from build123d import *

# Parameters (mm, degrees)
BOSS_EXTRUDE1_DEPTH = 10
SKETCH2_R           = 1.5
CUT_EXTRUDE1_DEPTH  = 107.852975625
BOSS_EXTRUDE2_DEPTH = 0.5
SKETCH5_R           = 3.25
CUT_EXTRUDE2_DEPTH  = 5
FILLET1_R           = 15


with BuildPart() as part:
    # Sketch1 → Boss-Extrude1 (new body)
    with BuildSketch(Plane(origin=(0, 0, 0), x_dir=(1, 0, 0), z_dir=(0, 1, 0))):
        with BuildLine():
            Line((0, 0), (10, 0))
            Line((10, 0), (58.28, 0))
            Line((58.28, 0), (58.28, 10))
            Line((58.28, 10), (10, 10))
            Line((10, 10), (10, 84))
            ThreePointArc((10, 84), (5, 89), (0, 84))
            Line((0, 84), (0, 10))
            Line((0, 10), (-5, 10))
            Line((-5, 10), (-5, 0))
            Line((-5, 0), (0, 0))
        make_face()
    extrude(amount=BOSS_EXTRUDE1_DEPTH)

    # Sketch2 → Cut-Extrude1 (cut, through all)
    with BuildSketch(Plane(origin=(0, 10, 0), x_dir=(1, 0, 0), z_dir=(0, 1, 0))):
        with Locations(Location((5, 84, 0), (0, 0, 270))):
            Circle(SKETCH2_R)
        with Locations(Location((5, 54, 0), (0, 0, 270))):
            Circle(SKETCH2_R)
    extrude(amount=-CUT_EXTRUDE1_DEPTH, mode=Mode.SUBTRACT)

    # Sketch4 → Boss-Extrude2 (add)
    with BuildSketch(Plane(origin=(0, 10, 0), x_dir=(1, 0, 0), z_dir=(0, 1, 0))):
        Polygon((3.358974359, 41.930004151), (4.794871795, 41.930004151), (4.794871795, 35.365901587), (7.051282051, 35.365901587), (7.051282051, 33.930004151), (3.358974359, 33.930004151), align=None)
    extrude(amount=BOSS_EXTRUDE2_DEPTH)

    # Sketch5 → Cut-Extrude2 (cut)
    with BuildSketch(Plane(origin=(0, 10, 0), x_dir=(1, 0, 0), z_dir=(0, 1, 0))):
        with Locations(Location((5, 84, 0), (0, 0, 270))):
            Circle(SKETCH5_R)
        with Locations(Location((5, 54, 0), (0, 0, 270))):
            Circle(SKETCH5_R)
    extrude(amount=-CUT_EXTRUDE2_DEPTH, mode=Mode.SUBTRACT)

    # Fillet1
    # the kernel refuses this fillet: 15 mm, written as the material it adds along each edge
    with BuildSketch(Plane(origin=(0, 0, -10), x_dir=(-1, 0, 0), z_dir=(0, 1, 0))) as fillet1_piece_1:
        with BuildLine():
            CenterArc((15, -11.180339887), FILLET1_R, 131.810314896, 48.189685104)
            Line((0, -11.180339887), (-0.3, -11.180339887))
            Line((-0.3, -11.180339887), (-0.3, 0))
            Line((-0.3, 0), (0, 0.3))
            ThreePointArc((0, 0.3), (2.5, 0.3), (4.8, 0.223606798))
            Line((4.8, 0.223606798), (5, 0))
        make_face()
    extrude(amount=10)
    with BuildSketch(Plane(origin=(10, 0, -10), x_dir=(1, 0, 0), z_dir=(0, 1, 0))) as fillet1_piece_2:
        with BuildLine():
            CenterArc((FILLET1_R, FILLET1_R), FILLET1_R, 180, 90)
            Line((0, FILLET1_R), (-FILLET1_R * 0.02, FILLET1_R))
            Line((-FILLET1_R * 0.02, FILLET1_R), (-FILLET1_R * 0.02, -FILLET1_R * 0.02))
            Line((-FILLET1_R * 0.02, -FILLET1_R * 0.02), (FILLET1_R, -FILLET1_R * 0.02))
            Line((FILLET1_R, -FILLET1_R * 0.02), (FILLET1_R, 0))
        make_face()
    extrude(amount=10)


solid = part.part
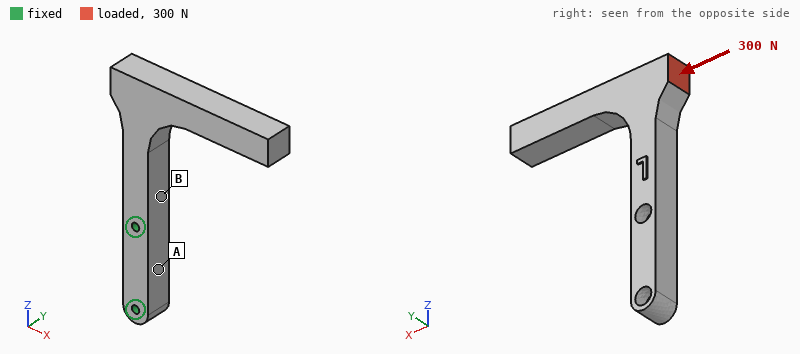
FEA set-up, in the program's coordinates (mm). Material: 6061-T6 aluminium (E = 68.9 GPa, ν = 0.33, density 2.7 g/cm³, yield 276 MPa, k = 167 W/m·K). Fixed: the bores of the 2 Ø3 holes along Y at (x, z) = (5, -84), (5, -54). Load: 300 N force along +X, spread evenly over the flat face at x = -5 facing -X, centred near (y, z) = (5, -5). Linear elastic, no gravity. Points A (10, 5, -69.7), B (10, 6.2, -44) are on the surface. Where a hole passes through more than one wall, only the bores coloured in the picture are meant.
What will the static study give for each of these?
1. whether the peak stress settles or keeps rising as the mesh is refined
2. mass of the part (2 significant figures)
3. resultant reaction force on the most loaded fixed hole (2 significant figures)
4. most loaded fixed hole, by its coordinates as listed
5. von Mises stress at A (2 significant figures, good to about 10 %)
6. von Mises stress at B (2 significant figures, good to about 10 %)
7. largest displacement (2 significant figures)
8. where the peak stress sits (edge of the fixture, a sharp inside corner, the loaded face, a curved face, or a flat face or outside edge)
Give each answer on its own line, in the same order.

keeps rising
39 g
620 N
(5, -54)
20 MPa
70 MPa
0.53 mm
edge of the fixture
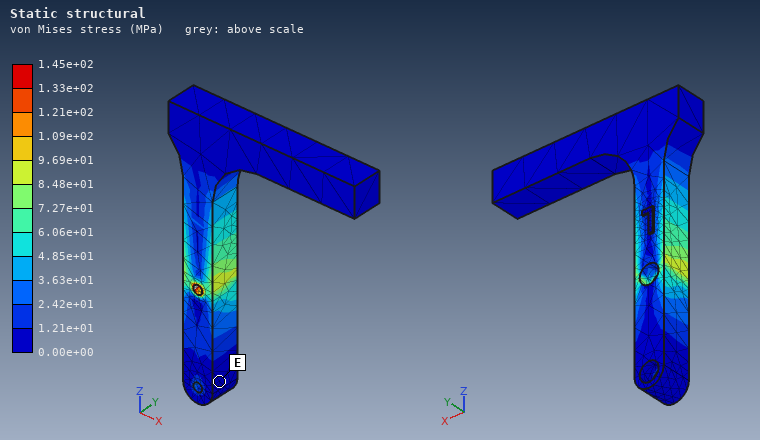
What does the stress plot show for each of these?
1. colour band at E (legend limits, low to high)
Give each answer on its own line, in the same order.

0.00e+00 to 1.21e+01 MPa
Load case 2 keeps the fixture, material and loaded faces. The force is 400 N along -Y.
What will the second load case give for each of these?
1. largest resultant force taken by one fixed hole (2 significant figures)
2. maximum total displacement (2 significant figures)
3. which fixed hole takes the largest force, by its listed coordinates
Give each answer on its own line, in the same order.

1.1 kN
0.52 mm
(5, -54)
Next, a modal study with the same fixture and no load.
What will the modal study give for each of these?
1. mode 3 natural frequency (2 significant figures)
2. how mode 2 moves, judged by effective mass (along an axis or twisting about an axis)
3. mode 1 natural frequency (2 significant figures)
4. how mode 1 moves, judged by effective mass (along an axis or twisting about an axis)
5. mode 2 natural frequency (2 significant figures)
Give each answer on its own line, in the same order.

2000 Hz
along X
860 Hz
along Y
910 Hz
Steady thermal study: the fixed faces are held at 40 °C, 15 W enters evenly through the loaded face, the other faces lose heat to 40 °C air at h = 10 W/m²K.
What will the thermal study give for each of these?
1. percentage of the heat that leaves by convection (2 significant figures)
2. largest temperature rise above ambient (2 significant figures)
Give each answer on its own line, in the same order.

8.6 %
44 K
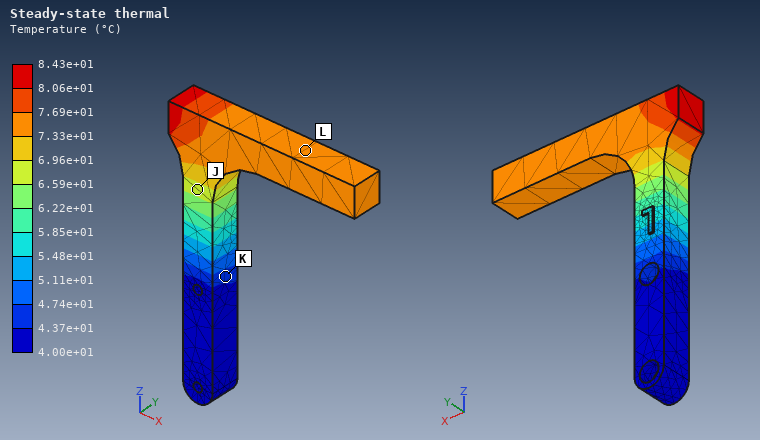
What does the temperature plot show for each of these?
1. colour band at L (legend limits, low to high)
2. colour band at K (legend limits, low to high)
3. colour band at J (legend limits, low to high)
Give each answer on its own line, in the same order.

7.33e+01 to 7.69e+01 °C
4.37e+01 to 4.74e+01 °C
6.59e+01 to 6.96e+01 °C
